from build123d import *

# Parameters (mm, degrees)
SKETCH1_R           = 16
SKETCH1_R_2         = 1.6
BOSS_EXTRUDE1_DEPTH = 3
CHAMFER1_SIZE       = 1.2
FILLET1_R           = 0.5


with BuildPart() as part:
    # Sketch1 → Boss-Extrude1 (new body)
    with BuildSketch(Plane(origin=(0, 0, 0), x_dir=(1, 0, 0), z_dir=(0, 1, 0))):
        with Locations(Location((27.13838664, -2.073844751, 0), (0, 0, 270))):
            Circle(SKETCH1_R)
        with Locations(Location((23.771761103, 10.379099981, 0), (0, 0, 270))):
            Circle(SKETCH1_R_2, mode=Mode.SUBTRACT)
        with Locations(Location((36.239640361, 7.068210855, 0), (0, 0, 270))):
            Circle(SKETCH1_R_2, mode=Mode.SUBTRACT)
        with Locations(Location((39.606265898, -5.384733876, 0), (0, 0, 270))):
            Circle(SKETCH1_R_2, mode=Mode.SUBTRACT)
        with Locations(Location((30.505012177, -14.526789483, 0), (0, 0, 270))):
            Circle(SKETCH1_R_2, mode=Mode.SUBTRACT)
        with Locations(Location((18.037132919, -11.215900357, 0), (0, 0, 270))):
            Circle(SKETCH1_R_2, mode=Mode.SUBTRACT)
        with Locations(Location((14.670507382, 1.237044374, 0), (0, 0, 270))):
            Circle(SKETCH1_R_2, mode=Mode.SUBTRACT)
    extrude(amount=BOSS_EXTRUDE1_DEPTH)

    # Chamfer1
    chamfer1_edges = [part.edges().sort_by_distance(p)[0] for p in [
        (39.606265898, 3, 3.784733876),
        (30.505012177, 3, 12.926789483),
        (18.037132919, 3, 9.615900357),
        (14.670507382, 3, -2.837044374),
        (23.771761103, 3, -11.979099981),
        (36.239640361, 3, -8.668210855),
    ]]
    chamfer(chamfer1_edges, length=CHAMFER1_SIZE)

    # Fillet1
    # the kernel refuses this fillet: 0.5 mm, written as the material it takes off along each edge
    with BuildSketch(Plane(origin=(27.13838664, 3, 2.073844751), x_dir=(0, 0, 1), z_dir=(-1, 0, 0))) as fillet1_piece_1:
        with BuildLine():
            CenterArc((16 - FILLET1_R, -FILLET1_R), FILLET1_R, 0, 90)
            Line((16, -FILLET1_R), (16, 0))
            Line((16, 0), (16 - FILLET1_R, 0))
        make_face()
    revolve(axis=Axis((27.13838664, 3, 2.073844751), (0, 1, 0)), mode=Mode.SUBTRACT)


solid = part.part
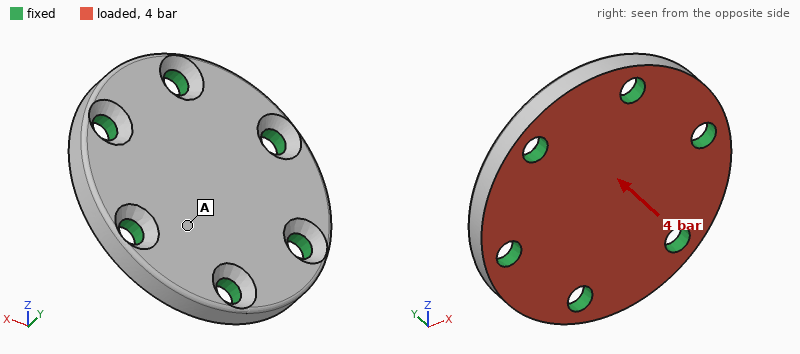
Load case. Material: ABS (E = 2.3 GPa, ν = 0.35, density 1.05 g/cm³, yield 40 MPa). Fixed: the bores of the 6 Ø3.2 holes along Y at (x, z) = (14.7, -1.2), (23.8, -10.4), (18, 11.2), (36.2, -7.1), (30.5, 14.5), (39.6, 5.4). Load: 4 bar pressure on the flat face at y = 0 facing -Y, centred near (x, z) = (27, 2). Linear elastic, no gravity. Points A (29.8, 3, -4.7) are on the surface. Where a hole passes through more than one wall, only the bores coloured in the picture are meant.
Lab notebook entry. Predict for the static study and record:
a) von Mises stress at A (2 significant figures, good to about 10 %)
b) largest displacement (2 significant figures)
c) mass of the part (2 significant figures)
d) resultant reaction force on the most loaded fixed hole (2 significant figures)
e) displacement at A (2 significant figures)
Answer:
2.8 MPa
43 µm
2.3 g
52 N
25 µm
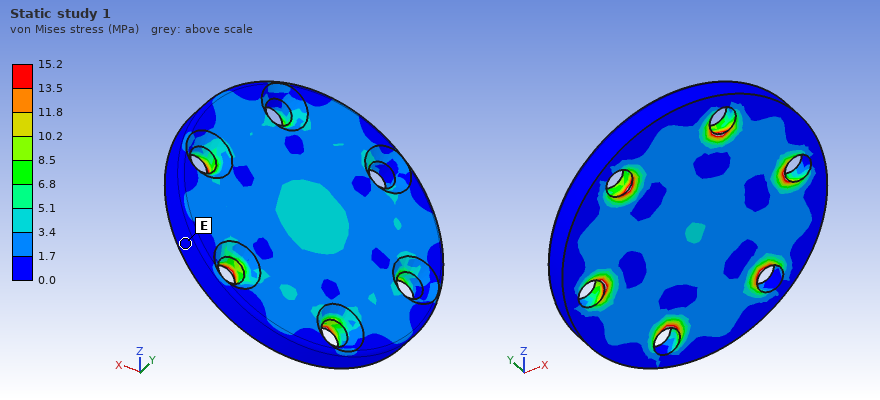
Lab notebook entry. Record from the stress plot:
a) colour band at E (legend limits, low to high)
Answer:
0.0 to 1.7 MPa
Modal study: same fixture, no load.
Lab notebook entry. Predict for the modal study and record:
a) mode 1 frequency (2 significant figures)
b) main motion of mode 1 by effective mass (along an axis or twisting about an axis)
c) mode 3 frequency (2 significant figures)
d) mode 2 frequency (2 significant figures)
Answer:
10 kHz
along Y
19 kHz
18 kHz
